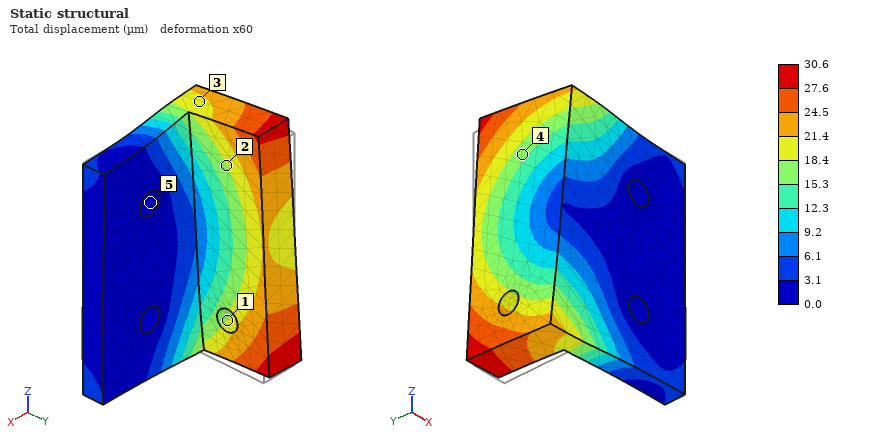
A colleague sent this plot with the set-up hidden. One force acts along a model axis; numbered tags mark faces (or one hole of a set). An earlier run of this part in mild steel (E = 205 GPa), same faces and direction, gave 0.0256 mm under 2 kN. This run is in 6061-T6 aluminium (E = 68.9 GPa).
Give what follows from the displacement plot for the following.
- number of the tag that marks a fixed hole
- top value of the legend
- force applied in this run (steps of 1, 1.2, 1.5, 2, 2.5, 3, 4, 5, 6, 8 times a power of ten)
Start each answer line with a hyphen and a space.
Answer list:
- 5
- 30.6 µm
- 800 N
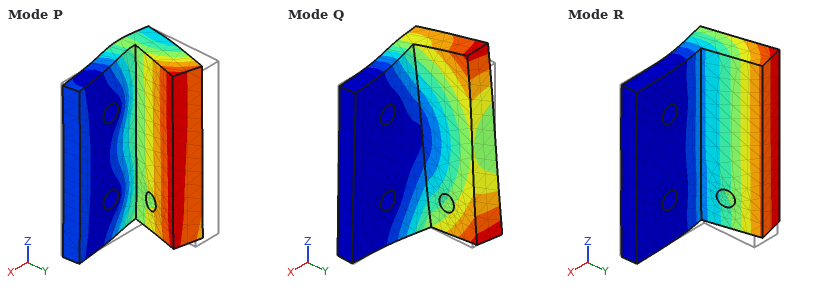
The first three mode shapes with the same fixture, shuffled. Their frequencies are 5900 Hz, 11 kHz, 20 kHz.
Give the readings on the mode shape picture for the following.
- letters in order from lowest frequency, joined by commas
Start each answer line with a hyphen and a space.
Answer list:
- R, Q, P
